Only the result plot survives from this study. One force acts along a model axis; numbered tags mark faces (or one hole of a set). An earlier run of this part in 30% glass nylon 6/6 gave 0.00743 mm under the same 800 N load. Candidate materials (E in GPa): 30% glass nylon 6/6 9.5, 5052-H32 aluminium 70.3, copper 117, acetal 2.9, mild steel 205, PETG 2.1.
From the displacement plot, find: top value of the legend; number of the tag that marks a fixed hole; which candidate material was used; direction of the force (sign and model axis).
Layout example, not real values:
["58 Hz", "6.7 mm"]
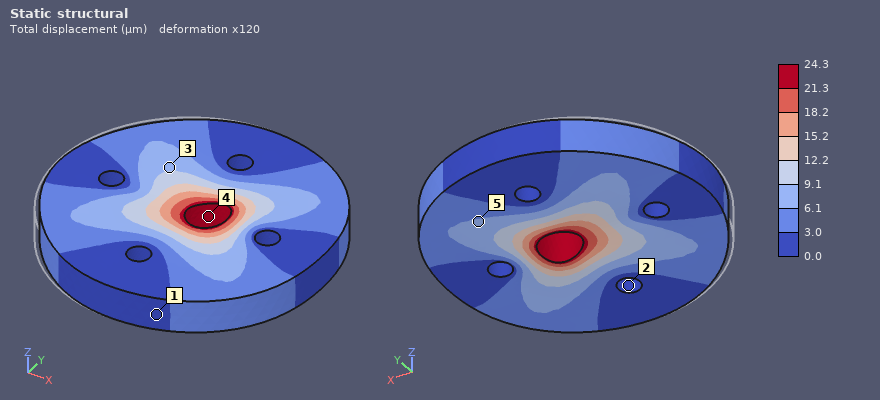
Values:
["24.3 µm", "2", "acetal", "+X"]
